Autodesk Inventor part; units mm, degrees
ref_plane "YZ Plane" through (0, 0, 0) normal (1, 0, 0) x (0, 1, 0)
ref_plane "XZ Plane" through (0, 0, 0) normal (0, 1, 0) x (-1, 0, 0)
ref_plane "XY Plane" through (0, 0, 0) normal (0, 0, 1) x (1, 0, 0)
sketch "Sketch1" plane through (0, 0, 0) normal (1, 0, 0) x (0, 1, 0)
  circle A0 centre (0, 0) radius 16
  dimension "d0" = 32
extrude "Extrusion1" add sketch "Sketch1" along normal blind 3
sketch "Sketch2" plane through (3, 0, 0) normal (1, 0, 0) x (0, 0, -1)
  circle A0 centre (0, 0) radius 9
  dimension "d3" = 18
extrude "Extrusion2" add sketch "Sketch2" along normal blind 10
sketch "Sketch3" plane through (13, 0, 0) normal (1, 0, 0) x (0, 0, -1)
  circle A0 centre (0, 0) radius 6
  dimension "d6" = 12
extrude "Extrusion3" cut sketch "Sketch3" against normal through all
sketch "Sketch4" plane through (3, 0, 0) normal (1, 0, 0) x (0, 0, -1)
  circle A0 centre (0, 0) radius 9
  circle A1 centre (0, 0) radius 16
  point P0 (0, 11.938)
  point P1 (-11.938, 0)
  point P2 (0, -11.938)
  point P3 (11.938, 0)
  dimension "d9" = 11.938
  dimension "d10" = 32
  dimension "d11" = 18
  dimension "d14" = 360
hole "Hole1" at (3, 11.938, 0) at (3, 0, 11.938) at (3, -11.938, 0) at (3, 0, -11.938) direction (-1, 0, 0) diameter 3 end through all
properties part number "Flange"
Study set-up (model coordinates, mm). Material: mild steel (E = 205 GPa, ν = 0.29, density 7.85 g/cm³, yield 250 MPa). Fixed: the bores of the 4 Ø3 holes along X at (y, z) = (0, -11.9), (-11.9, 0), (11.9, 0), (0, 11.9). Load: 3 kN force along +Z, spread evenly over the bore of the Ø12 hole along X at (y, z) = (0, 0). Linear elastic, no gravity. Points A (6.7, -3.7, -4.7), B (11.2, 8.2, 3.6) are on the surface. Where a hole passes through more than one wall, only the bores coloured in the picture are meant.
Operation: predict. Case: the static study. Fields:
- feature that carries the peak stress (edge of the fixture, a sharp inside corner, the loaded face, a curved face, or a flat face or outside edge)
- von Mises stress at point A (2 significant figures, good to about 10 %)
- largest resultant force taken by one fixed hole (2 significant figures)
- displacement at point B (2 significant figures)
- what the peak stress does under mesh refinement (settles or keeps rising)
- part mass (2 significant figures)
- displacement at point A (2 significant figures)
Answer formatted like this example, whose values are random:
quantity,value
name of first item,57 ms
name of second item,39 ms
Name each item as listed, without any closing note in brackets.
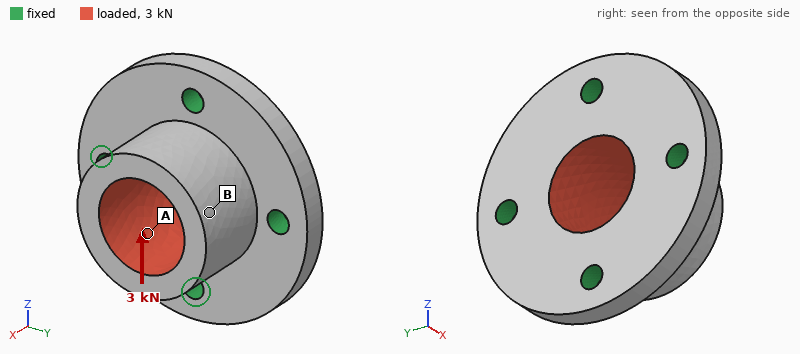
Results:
quantity,value
feature that carries the peak stress,edge of the fixture
von Mises stress at point A,32 MPa
largest resultant force taken by one fixed hole,1.1 kN
displacement at point B,4.4 µm
what the peak stress does under mesh refinement,keeps rising
part mass,27 g
displacement at point A,2.9 µm
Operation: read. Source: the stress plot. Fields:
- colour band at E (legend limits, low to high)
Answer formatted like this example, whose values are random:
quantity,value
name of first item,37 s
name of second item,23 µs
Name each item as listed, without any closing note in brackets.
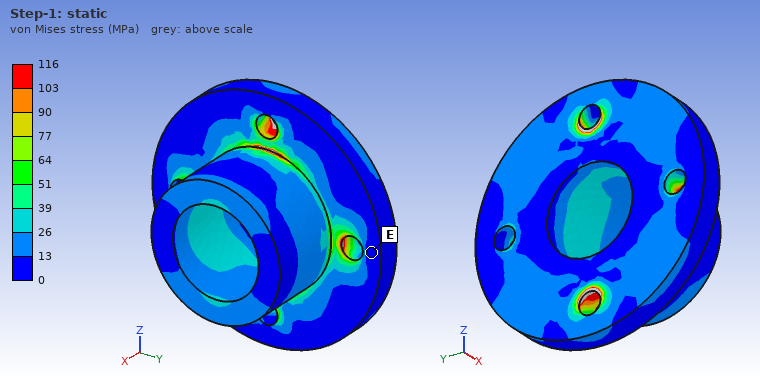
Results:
quantity,value
colour band at E,0 to 13 MPa
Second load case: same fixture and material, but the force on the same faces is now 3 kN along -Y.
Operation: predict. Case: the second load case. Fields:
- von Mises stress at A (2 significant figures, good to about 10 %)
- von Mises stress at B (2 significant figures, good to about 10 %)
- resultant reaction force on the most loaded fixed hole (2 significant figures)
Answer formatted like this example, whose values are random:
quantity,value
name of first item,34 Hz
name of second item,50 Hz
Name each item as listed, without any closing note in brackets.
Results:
quantity,value
von Mises stress at A,35 MPa
von Mises stress at B,13 MPa
resultant reaction force on the most loaded fixed hole,1.1 kN
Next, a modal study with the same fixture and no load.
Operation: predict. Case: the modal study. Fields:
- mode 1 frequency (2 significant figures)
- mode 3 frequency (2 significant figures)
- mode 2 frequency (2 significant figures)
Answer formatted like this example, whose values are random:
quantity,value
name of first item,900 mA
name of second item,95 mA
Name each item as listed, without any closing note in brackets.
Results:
quantity,value
mode 1 frequency,32 kHz
mode 3 frequency,36 kHz
mode 2 frequency,32 kHz
